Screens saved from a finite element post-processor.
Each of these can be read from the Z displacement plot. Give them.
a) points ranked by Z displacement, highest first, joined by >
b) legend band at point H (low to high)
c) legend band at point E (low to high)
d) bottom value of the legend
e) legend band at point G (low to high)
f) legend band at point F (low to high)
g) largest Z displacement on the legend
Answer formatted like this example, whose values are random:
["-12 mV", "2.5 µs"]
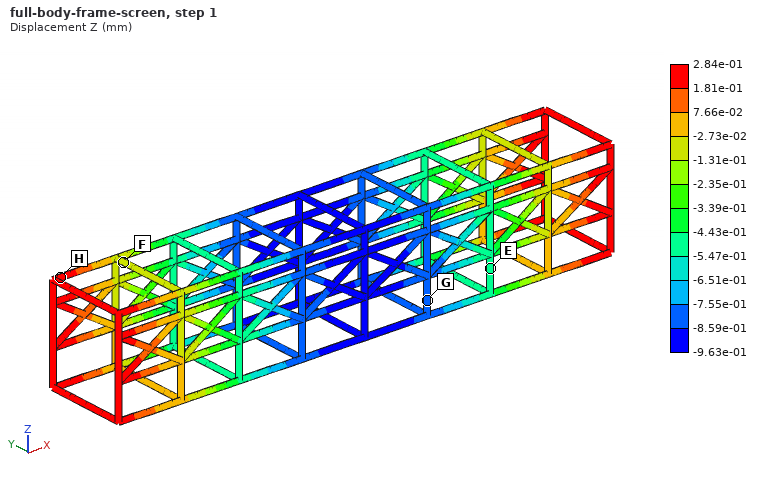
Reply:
["H > F > E > G", "1.81e-01 to 2.84e-01 mm", "-5.47e-01 to -4.43e-01 mm", "-9.63e-01 mm", "-8.59e-01 to -7.55e-01 mm", "-1.31e-01 to -2.73e-02 mm", "2.84e-01 mm"]
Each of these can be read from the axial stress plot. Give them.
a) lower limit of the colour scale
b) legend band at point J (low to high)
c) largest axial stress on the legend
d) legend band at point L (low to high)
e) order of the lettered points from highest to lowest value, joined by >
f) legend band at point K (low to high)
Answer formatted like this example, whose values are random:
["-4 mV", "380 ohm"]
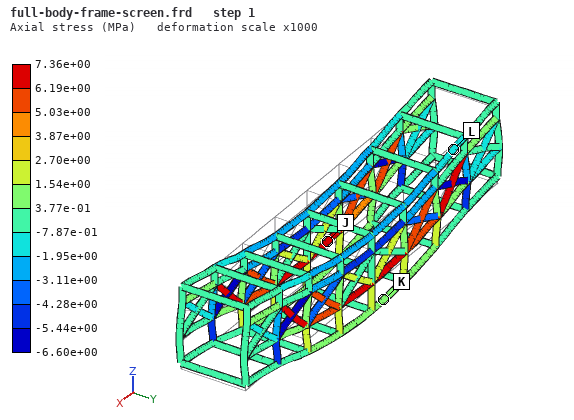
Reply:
["-6.60e+00 MPa", "6.19e+00 to 7.36e+00 MPa", "7.36e+00 MPa", "-1.95e+00 to -7.87e-01 MPa", "J > K > L", "3.77e-01 to 1.54e+00 MPa"]
